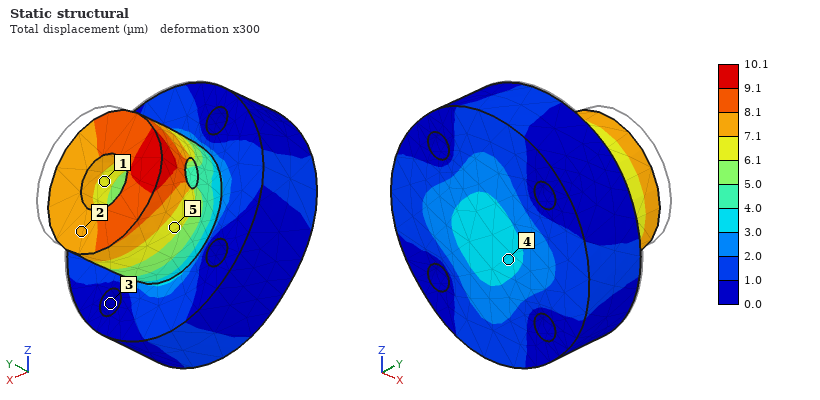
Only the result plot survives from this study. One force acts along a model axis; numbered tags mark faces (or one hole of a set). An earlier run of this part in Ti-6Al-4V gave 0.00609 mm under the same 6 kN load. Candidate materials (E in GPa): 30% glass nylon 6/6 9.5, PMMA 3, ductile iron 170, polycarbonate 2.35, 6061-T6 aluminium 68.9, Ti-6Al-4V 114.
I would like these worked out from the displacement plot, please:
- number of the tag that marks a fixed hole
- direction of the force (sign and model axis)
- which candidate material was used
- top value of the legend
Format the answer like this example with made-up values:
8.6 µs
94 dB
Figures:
3
-Y
6061-T6 aluminium
10.1 µm
